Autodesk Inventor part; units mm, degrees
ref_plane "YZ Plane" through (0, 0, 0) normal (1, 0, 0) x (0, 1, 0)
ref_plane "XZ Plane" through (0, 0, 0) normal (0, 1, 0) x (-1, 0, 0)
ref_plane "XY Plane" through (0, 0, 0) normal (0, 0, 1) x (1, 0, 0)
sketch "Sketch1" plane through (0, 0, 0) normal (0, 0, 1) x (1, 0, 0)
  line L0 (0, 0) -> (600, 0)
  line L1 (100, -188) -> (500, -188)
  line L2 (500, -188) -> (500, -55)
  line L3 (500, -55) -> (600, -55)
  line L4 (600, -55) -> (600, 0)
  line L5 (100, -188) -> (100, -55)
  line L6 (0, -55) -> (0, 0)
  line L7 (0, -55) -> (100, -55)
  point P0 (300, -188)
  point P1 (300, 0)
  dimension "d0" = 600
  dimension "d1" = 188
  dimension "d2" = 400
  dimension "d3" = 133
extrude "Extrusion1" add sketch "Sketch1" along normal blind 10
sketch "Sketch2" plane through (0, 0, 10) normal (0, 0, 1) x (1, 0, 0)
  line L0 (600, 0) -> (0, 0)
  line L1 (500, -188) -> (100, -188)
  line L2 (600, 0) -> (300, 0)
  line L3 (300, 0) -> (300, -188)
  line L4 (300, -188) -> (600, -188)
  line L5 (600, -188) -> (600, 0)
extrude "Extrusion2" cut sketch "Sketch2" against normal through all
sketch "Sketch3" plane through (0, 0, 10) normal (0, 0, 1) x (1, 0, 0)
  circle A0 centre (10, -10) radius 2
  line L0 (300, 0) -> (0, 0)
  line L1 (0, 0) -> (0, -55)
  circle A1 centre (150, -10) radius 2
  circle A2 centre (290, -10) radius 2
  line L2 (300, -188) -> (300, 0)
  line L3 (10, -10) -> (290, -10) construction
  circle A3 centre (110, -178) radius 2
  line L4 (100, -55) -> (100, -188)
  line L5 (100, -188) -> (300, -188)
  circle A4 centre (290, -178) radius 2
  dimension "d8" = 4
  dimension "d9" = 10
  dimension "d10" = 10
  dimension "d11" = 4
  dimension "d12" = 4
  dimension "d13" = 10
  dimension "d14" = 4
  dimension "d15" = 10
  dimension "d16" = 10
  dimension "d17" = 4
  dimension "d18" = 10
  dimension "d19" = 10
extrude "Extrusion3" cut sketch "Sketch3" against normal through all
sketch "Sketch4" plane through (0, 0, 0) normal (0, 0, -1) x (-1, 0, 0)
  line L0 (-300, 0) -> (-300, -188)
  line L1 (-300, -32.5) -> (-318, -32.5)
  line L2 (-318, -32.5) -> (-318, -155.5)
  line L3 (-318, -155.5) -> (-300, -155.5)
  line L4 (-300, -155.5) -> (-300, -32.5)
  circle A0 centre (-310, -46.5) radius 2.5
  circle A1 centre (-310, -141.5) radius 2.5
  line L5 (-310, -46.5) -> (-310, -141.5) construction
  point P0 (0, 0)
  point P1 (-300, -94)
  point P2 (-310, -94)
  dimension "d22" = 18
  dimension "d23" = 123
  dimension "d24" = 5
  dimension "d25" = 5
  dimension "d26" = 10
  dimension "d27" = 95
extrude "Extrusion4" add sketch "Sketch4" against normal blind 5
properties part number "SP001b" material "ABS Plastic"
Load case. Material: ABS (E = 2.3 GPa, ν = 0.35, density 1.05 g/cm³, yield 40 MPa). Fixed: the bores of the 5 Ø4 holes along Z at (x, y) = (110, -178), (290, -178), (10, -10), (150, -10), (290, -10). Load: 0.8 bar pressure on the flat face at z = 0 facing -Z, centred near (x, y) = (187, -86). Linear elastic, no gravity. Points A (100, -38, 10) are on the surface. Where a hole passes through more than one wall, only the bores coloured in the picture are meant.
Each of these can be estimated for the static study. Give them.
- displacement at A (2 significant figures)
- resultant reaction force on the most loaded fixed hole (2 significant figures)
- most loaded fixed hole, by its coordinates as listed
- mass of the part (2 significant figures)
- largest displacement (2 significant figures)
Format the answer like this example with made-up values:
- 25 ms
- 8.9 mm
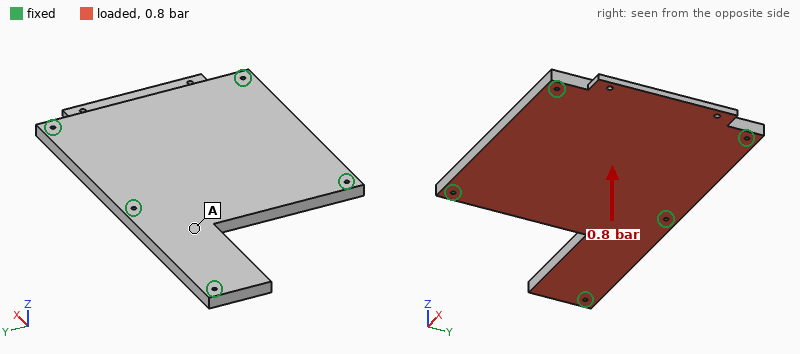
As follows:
- 1.1 mm
- 1.1 kN
- (150, -10)
- 460 g
- 2.9 mm
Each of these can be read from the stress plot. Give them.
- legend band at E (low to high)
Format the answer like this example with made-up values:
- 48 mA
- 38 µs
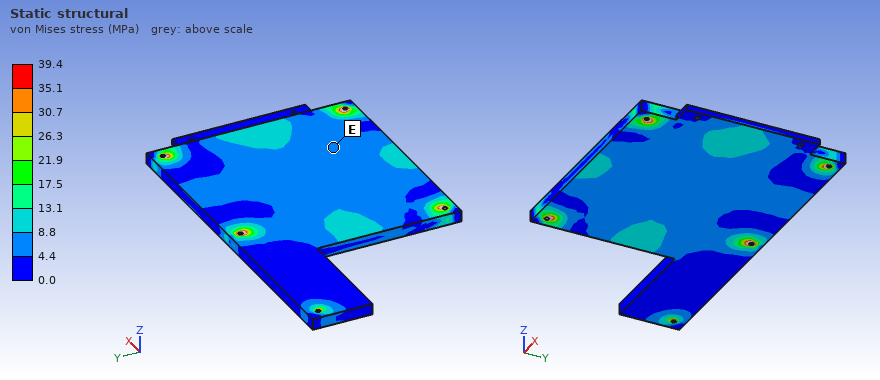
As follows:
- 4.4 to 8.8 MPa
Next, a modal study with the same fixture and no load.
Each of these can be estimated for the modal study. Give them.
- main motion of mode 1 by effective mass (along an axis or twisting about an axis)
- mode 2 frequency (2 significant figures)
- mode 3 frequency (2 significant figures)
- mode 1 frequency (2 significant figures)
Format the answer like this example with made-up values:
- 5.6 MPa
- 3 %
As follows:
- along Z
- 450 Hz
- 480 Hz
- 310 Hz
